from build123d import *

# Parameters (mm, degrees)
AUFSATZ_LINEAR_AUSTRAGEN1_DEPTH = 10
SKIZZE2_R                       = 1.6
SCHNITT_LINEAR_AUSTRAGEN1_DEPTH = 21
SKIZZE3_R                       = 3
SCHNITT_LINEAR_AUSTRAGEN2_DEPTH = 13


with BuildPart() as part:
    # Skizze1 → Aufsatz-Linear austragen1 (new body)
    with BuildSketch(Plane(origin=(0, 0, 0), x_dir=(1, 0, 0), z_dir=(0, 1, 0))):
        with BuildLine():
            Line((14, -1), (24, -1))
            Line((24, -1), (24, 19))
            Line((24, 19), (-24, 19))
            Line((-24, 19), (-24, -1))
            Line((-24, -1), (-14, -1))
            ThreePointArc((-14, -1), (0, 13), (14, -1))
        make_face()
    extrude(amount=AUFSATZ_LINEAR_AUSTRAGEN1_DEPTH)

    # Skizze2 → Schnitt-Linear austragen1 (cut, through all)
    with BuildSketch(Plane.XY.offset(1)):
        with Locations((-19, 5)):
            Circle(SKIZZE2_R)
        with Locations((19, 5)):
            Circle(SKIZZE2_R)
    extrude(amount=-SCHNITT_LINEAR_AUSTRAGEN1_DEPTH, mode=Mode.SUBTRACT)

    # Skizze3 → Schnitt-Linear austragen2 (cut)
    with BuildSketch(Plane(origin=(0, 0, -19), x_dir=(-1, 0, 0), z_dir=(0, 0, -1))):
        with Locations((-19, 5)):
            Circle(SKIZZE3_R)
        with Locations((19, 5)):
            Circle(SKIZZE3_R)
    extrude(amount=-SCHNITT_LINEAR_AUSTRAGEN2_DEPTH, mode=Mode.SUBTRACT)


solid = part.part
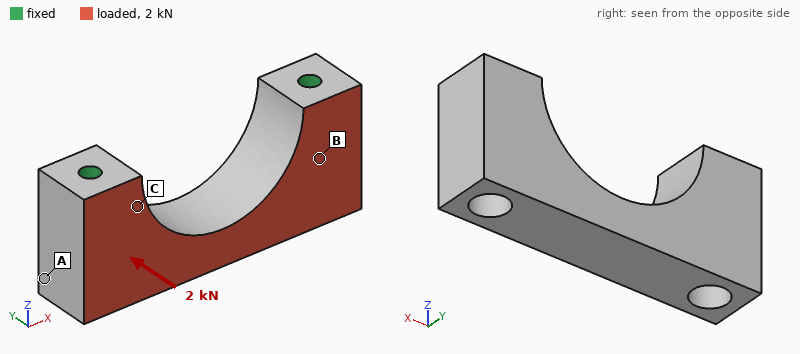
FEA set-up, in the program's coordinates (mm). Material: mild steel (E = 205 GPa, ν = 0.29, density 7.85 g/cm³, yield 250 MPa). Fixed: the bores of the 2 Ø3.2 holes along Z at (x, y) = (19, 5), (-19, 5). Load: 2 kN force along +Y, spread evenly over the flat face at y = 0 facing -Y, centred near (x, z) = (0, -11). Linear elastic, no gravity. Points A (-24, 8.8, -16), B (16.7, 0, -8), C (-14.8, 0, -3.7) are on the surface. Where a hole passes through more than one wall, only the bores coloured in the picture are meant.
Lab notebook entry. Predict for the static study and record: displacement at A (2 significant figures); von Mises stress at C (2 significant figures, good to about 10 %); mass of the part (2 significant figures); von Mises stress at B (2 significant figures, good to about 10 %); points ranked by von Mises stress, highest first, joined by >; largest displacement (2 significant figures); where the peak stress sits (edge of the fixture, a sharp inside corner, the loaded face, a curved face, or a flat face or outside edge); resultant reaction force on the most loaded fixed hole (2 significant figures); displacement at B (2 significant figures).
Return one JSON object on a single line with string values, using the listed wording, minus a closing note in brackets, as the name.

{"displacement at A": "6.0 µm", "von Mises stress at C": "39 MPa", "mass of the part": "45 g", "von Mises stress at B": "22 MPa", "points ranked by von Mises stress, highest first, joined by >": "C > B > A", "largest displacement": "12 µm", "where the peak stress sits": "edge of the fixture", "resultant reaction force on the most loaded fixed hole": "1.0 kN", "displacement at B": "3.7 µm"}
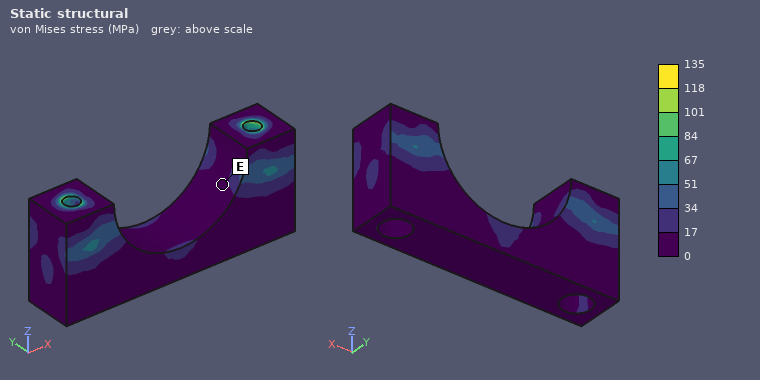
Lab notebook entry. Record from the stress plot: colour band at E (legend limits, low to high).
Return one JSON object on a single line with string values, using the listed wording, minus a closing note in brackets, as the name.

{"colour band at E": "0 to 17 MPa"}
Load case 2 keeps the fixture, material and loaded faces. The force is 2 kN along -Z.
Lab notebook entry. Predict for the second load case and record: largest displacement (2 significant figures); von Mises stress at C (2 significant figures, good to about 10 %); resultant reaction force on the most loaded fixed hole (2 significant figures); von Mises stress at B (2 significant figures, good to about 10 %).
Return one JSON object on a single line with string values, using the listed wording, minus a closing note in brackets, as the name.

{"largest displacement": "6.7 µm", "von Mises stress at C": "25 MPa", "resultant reaction force on the most loaded fixed hole": "1.0 kN", "von Mises stress at B": "26 MPa"}
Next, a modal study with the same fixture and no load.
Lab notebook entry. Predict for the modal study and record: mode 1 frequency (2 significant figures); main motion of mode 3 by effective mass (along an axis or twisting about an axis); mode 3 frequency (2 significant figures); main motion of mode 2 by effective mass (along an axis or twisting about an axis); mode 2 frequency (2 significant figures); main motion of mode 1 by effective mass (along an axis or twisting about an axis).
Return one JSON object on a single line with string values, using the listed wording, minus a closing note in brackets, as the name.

{"mode 1 frequency": "12 kHz", "main motion of mode 3 by effective mass": "along X", "mode 3 frequency": "22 kHz", "main motion of mode 2 by effective mass": "twisting about Z", "mode 2 frequency": "21 kHz", "main motion of mode 1 by effective mass": "along Y"}
